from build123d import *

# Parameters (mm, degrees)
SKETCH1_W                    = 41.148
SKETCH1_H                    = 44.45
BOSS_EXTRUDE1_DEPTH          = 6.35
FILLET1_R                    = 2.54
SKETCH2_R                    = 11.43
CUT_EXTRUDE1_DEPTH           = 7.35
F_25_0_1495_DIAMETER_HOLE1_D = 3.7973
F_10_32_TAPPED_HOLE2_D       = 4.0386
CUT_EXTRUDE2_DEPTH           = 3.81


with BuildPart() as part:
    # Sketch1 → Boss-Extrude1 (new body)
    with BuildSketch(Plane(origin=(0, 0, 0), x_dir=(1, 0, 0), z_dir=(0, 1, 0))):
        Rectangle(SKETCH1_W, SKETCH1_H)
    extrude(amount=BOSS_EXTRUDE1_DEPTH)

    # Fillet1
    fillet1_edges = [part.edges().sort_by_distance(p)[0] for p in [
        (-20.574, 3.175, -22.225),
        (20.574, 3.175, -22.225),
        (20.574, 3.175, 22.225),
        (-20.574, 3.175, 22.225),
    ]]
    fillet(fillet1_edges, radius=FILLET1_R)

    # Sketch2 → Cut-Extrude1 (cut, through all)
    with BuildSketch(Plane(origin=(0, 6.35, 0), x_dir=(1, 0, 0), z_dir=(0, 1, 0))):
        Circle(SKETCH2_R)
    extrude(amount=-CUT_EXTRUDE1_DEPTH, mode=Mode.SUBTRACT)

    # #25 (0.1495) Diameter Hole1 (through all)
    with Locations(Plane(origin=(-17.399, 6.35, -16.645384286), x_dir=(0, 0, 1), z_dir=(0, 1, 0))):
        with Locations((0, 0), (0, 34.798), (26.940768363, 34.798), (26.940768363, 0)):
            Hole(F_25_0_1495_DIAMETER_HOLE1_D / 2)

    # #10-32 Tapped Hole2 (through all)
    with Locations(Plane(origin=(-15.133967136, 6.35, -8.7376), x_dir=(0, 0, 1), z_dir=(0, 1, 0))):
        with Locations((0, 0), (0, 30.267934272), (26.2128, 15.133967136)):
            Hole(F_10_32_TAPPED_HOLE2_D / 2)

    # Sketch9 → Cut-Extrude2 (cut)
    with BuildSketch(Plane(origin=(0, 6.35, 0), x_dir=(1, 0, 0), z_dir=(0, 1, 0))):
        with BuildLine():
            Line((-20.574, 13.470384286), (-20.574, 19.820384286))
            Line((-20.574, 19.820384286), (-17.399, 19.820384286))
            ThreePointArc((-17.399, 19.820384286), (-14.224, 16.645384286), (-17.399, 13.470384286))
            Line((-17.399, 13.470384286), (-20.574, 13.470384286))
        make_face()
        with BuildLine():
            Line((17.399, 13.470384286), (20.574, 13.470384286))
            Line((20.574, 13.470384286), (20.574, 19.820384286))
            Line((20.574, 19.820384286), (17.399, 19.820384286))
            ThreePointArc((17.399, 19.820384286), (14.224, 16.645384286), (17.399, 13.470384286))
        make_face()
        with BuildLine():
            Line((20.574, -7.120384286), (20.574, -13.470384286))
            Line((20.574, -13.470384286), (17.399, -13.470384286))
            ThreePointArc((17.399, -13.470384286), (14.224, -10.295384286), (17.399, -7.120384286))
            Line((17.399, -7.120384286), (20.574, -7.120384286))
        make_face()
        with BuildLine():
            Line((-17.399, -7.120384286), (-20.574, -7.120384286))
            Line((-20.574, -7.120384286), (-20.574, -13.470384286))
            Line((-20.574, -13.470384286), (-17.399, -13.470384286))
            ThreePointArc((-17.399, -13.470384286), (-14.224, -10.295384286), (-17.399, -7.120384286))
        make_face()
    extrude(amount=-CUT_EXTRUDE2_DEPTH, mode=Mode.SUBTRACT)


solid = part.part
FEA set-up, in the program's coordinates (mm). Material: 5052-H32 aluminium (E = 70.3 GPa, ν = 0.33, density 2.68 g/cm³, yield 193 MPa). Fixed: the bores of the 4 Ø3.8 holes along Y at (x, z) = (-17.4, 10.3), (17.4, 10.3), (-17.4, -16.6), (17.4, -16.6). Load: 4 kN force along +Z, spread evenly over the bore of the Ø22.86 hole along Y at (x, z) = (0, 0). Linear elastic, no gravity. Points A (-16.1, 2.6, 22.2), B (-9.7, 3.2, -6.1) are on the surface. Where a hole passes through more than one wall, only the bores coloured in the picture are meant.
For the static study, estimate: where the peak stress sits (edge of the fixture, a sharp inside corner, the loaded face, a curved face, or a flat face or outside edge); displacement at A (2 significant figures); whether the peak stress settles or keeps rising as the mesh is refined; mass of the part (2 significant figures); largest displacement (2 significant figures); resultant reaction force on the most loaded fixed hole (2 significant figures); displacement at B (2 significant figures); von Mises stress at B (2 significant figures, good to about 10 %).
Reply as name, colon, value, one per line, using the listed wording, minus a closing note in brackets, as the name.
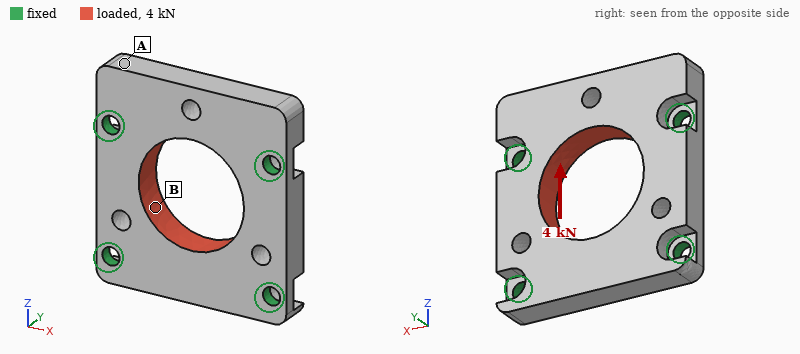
where the peak stress sits: edge of the fixture
displacement at A: 8.4 µm
whether the peak stress settles or keeps rising as the mesh is refined: keeps rising
mass of the part: 22 g
largest displacement: 13 µm
resultant reaction force on the most loaded fixed hole: 1.2 kN
displacement at B: 5.1 µm
von Mises stress at B: 25 MPa
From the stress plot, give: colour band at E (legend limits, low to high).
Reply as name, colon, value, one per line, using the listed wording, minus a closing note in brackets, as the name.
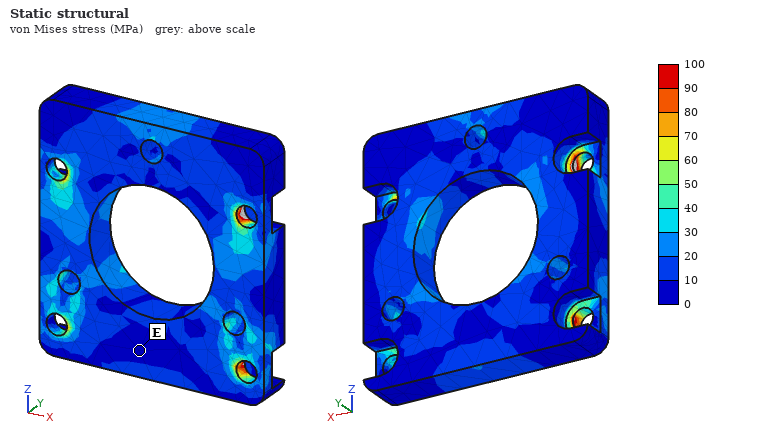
colour band at E: 0 to 10 MPa
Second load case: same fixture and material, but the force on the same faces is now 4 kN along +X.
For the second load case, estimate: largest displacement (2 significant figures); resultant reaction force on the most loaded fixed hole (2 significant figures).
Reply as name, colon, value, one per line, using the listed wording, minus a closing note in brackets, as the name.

largest displacement: 8.9 µm
resultant reaction force on the most loaded fixed hole: 1.1 kN
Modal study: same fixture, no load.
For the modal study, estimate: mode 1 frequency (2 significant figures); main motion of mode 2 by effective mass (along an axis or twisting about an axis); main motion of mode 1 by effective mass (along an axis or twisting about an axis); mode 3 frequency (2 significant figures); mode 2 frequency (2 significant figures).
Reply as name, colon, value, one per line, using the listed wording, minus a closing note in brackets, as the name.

mode 1 frequency: 12 kHz
main motion of mode 2 by effective mass: along Y
main motion of mode 1 by effective mass: along Y
mode 3 frequency: 23 kHz
mode 2 frequency: 18 kHz
